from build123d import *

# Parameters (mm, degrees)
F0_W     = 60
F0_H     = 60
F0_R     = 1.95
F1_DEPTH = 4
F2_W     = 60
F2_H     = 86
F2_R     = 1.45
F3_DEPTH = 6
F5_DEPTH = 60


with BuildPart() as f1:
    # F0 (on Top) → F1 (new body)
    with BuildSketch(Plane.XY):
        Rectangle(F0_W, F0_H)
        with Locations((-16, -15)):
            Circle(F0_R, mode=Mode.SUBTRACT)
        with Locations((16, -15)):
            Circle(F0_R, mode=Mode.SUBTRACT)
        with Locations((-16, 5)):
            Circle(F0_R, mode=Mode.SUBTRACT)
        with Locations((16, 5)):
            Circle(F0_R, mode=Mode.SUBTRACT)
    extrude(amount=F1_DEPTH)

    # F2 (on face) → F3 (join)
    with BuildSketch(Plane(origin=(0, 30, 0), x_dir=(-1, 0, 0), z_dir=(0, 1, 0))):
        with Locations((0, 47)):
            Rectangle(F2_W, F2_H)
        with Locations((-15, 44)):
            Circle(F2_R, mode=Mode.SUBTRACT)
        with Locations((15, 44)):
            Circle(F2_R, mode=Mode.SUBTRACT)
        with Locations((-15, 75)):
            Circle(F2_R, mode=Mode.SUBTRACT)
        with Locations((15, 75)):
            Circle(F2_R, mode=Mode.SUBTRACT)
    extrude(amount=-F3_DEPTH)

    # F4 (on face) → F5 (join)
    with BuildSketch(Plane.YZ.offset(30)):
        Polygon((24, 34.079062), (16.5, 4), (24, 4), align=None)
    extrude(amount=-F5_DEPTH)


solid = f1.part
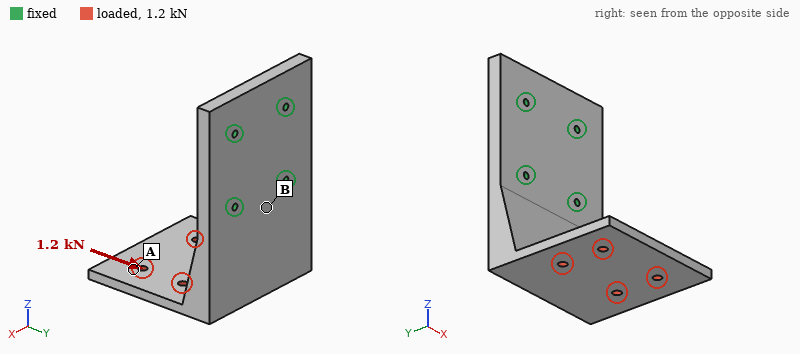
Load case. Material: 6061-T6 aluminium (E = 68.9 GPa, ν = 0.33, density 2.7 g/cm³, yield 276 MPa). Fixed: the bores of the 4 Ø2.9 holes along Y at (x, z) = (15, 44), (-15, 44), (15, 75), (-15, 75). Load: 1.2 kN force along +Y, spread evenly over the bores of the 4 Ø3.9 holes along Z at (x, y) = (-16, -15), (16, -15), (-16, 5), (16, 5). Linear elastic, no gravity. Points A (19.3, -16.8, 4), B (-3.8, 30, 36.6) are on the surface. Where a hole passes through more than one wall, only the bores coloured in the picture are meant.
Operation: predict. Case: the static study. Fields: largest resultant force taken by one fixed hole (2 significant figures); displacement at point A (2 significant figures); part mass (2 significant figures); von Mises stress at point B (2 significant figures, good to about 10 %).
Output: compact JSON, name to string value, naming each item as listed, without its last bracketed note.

{"largest resultant force taken by one fixed hole": "970 N", "displacement at point A": "0.60 mm", "part mass": "140 g", "von Mises stress at point B": "93 MPa"}
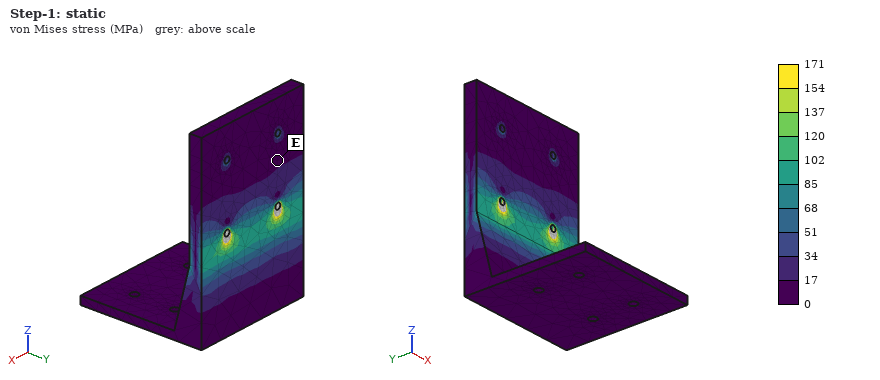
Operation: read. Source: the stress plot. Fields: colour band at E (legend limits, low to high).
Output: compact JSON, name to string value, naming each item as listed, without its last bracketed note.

{"colour band at E": "0 to 17 MPa"}
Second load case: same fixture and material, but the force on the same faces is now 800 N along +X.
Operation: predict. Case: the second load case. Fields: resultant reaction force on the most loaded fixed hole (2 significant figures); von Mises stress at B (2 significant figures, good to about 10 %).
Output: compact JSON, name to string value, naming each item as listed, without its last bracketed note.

{"resultant reaction force on the most loaded fixed hole": "1.1 kN", "von Mises stress at B": "15 MPa"}
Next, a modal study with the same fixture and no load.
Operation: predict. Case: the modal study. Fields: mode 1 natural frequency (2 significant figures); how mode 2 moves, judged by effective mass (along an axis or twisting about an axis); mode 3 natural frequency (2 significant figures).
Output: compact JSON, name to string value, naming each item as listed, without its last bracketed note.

{"mode 1 natural frequency": "860 Hz", "how mode 2 moves, judged by effective mass": "along Y", "mode 3 natural frequency": "2000 Hz"}
